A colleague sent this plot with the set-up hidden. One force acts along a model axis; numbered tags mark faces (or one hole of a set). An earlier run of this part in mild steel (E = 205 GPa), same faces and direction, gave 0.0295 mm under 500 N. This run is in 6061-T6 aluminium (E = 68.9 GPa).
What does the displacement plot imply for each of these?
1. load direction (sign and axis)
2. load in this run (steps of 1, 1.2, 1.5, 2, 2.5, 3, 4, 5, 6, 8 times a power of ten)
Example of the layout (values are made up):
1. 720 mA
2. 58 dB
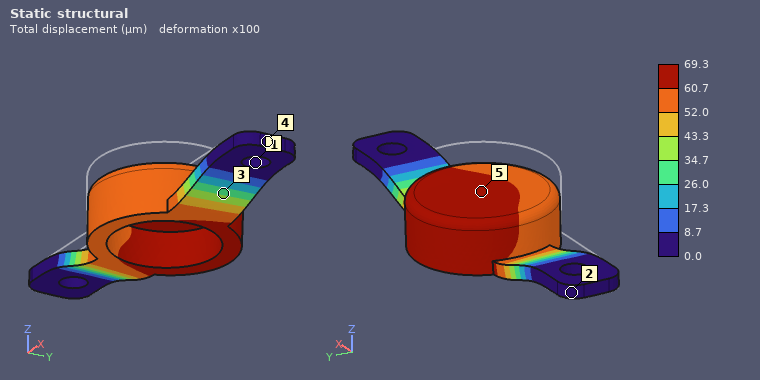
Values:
1. -Z
2. 400 N
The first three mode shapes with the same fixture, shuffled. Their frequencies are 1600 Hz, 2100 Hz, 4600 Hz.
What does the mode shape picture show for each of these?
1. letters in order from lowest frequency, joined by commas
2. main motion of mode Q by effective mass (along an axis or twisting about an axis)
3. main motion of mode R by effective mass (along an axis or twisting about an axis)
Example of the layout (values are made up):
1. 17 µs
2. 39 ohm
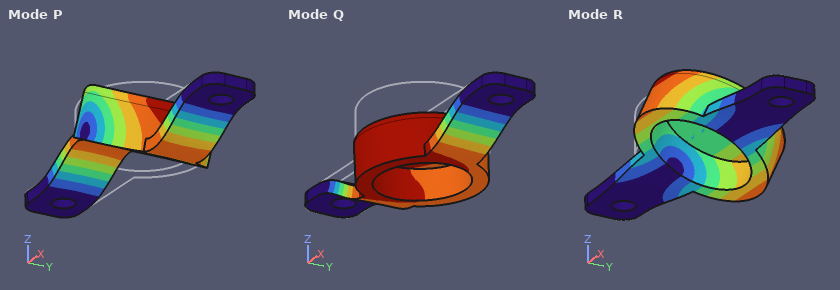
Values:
1. R, Q, P
2. along Z
3. along Y
